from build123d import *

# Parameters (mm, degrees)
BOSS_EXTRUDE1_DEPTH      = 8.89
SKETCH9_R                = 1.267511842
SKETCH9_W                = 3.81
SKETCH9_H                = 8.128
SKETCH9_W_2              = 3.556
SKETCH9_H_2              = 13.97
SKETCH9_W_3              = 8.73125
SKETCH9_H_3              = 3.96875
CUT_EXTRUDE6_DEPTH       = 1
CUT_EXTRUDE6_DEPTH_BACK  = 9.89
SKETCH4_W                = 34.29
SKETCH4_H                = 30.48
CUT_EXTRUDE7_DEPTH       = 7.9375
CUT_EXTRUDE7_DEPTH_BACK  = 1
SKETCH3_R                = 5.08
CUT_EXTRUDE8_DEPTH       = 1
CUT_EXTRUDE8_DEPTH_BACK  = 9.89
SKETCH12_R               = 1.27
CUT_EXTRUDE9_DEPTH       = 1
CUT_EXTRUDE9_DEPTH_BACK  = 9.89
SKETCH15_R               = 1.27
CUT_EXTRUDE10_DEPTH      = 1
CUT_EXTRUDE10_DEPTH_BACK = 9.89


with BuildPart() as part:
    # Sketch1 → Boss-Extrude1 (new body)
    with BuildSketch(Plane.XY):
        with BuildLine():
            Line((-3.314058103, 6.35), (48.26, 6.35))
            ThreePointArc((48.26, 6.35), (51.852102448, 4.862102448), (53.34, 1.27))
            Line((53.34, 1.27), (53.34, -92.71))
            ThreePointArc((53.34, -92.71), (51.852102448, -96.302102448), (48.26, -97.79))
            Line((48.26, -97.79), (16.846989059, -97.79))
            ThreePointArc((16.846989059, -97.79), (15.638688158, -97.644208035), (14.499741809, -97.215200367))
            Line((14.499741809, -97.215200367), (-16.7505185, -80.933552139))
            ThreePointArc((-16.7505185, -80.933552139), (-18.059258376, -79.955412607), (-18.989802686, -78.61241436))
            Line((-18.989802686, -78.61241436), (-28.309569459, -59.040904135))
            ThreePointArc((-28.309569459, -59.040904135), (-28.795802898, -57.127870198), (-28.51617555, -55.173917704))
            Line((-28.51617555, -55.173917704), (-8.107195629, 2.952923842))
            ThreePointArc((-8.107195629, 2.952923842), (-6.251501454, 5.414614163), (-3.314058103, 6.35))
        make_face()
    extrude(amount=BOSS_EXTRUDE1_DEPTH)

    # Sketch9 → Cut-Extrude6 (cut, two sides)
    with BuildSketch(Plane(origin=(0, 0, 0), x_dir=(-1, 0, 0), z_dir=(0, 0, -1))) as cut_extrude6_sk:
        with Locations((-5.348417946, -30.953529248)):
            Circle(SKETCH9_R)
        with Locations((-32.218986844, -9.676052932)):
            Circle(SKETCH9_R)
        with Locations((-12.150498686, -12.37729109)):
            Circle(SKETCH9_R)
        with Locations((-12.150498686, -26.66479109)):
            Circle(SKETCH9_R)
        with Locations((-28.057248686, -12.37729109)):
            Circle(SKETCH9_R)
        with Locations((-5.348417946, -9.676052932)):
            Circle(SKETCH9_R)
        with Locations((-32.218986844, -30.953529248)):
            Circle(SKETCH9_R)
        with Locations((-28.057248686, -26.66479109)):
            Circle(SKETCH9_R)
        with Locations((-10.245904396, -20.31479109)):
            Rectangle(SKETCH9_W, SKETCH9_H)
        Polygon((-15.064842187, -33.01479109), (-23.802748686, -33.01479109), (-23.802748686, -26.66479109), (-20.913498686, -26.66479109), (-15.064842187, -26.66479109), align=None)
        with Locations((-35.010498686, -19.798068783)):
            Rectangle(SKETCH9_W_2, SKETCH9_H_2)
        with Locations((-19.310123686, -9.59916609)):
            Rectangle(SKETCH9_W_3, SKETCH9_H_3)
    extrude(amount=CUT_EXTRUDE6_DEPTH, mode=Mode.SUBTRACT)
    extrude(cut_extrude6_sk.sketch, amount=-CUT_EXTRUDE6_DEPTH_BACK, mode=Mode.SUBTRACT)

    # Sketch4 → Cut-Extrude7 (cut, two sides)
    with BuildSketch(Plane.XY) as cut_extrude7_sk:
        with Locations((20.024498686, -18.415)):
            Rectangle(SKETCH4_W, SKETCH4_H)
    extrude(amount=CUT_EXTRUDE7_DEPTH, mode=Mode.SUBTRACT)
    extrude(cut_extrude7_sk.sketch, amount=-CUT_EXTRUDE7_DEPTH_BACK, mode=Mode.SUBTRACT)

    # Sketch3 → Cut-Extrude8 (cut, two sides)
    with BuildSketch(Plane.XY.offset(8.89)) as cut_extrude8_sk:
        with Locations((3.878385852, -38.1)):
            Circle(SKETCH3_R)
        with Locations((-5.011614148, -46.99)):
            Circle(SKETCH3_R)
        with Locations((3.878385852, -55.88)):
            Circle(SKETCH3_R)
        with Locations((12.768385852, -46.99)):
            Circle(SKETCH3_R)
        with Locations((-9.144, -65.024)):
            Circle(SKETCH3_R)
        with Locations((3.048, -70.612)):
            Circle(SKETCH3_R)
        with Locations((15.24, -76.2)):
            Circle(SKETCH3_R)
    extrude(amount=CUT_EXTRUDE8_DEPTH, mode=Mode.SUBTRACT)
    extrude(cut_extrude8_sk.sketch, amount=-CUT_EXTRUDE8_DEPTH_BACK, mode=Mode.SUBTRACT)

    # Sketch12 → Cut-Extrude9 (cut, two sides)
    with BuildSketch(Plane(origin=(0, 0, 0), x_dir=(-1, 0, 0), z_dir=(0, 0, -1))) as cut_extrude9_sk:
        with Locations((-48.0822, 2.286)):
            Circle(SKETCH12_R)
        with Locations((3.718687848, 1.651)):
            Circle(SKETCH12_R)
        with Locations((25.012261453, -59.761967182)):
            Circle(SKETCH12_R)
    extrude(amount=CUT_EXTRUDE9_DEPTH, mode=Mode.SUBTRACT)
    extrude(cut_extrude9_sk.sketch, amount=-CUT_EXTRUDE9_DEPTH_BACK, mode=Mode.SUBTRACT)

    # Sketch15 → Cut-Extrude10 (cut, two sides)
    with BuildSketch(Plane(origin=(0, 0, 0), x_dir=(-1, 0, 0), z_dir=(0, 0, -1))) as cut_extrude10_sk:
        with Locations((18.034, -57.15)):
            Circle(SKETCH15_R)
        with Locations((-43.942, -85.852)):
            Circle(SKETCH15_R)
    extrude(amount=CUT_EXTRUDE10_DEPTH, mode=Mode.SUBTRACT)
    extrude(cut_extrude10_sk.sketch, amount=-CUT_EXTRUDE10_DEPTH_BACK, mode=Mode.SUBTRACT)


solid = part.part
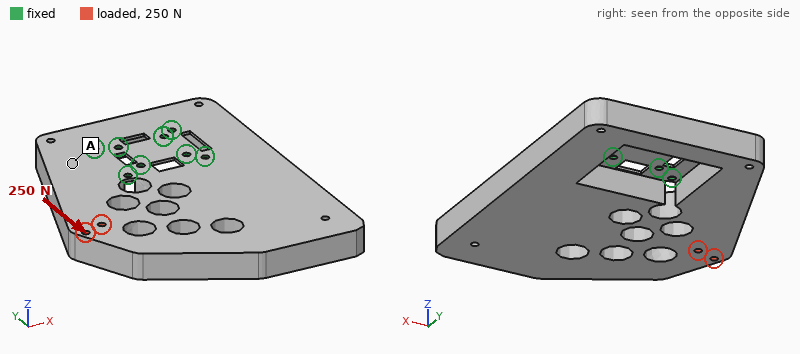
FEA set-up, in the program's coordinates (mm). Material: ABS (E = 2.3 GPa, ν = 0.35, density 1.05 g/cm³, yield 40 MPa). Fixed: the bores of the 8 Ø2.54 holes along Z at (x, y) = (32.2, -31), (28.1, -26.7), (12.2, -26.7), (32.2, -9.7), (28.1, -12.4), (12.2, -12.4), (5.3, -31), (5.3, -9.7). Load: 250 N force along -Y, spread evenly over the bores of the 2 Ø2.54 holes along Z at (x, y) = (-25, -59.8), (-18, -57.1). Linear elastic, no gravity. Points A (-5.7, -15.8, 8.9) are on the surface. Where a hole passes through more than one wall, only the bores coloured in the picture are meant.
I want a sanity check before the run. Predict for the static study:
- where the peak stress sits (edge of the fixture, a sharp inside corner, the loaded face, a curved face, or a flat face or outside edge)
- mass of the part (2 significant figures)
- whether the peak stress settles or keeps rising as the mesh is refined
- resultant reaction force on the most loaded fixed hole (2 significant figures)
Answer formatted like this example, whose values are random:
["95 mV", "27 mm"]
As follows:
["edge of the fixture", "53 g", "keeps rising", "200 N"]
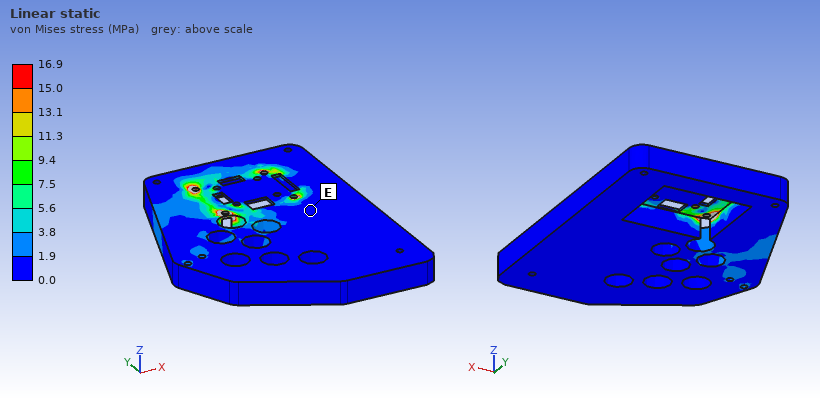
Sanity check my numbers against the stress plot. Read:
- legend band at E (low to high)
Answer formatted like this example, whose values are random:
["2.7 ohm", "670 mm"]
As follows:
["0.0 to 1.9 MPa"]
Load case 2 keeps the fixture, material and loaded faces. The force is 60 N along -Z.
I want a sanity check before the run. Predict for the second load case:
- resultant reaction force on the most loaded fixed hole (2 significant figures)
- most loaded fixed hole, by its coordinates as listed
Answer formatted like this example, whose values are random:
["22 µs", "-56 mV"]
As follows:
["150 N", "(5.3, -31)"]
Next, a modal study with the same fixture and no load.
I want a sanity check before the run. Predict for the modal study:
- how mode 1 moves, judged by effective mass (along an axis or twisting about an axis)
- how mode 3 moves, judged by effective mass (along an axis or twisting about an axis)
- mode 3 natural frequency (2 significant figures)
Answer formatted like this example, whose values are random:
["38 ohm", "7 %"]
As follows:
["along Z", "along X", "870 Hz"]
